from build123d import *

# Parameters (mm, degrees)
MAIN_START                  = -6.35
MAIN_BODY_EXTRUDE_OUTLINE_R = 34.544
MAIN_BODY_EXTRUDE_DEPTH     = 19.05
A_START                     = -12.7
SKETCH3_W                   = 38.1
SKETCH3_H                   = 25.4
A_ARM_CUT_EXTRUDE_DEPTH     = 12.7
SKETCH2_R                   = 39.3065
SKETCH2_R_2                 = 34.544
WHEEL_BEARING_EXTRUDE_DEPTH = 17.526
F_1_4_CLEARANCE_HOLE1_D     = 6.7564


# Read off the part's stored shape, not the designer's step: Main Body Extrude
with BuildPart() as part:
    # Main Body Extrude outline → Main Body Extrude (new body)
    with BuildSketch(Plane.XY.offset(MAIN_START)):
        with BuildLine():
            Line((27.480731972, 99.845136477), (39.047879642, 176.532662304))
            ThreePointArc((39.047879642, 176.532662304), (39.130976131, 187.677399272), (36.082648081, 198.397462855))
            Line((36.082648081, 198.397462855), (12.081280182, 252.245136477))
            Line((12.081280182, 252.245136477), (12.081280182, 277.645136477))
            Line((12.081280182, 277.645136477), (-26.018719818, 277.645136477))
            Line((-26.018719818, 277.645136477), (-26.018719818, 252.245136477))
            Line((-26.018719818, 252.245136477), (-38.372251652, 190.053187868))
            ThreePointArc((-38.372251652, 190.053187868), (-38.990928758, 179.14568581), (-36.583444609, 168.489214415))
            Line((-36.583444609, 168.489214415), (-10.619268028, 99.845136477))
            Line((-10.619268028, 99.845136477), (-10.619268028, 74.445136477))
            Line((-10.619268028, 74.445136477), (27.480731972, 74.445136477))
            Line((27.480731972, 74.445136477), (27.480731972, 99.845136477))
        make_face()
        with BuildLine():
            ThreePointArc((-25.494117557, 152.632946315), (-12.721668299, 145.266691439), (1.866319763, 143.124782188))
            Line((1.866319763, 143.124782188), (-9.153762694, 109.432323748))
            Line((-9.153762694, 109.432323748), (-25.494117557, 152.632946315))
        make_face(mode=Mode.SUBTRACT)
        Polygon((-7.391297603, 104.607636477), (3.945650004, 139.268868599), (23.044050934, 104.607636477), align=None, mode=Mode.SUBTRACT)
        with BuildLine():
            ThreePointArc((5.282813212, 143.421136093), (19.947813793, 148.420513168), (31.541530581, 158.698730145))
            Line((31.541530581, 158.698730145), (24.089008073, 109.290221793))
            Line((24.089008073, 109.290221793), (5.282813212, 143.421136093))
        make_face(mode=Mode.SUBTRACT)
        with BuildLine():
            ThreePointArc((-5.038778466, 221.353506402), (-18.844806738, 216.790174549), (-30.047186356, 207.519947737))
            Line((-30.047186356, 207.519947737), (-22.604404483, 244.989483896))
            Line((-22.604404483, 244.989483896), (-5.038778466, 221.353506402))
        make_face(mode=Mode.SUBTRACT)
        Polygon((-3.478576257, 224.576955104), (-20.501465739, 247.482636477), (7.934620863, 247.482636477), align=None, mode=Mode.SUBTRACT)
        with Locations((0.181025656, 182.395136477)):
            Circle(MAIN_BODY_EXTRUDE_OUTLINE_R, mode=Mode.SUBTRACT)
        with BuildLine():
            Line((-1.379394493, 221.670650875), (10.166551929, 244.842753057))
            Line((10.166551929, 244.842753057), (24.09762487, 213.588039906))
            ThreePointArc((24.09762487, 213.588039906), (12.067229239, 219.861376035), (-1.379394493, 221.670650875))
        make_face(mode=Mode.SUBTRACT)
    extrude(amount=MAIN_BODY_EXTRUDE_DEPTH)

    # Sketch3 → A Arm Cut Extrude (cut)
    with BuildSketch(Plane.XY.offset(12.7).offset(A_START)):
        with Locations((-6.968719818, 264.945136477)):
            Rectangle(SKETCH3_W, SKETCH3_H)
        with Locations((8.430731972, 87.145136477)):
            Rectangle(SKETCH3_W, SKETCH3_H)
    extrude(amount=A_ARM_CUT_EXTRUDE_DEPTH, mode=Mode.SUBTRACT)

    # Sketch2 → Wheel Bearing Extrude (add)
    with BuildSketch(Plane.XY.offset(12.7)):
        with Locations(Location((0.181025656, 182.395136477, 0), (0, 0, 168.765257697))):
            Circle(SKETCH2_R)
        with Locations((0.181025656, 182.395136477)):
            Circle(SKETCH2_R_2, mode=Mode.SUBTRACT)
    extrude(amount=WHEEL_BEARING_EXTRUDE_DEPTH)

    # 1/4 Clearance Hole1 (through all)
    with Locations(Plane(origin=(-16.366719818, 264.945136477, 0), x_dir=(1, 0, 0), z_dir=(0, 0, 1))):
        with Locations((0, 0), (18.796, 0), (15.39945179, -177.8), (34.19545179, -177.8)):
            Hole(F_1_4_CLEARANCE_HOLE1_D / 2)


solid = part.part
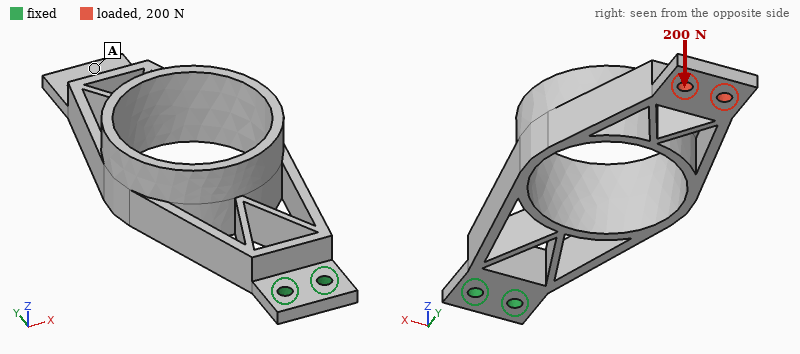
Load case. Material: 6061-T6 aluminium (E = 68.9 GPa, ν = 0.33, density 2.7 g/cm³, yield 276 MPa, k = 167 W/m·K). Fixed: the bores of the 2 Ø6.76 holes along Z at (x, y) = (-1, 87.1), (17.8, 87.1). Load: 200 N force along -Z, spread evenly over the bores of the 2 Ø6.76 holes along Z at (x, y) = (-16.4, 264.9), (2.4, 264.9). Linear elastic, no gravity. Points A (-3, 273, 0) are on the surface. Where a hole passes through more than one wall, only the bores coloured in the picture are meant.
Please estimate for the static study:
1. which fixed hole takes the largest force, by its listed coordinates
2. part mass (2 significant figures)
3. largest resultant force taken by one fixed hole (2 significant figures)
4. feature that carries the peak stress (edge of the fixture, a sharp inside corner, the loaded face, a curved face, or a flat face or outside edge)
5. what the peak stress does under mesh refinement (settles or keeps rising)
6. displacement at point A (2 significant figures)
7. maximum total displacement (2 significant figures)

(-1, 87.1)
230 g
290 N
edge of the fixture
keeps rising
2.5 mm
2.6 mm
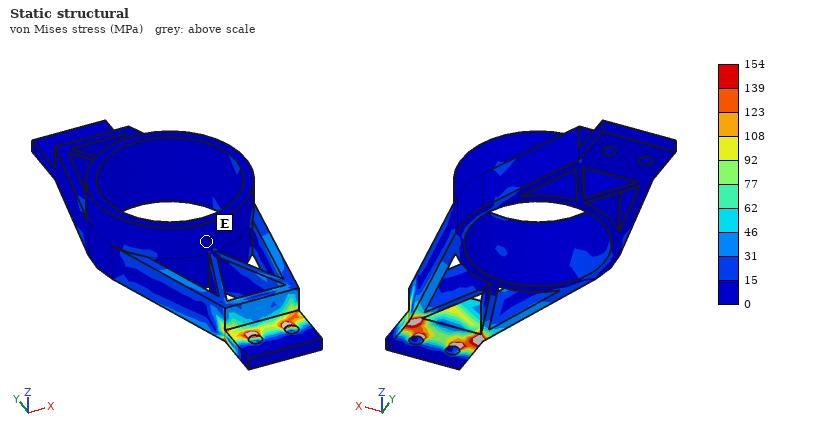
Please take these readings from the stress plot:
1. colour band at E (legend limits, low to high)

0 to 15 MPa
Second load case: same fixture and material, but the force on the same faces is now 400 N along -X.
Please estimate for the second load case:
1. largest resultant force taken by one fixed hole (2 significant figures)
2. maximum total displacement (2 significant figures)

3.0 kN
0.55 mm
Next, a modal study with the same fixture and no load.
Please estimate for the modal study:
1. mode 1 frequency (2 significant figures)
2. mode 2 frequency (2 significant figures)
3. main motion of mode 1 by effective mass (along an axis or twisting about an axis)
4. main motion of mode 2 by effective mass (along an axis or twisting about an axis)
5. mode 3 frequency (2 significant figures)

170 Hz
520 Hz
along Z
along X
860 Hz
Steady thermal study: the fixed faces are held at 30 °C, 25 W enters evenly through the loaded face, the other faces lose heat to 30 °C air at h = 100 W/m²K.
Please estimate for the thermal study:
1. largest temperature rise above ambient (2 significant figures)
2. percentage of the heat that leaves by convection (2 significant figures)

28 K
96 %
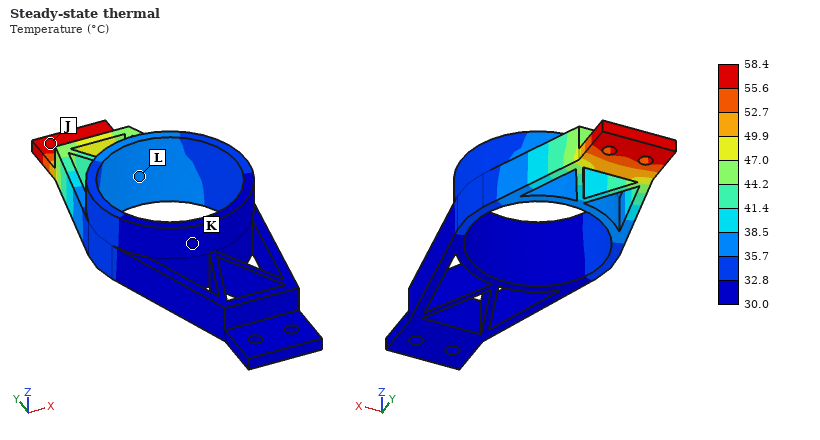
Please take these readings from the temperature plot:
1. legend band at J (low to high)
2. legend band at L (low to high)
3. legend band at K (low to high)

55.6 to 58.4 °C
35.7 to 38.5 °C
30.0 to 32.8 °C
